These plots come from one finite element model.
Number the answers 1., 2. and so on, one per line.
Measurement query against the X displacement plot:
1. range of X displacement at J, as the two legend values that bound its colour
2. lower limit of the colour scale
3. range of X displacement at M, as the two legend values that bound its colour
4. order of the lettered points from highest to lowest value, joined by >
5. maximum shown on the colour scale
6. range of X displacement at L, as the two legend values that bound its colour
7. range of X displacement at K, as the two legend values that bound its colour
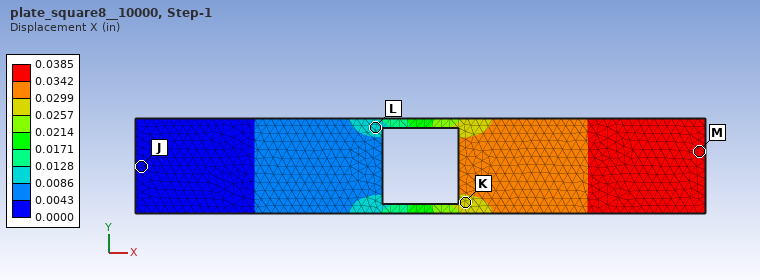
1. 0.0000 to 0.0043 in
2. 0.0000 in
3. 0.0342 to 0.0385 in
4. M > K > L > J
5. 0.0385 in
6. 0.0086 to 0.0128 in
7. 0.0257 to 0.0299 in
